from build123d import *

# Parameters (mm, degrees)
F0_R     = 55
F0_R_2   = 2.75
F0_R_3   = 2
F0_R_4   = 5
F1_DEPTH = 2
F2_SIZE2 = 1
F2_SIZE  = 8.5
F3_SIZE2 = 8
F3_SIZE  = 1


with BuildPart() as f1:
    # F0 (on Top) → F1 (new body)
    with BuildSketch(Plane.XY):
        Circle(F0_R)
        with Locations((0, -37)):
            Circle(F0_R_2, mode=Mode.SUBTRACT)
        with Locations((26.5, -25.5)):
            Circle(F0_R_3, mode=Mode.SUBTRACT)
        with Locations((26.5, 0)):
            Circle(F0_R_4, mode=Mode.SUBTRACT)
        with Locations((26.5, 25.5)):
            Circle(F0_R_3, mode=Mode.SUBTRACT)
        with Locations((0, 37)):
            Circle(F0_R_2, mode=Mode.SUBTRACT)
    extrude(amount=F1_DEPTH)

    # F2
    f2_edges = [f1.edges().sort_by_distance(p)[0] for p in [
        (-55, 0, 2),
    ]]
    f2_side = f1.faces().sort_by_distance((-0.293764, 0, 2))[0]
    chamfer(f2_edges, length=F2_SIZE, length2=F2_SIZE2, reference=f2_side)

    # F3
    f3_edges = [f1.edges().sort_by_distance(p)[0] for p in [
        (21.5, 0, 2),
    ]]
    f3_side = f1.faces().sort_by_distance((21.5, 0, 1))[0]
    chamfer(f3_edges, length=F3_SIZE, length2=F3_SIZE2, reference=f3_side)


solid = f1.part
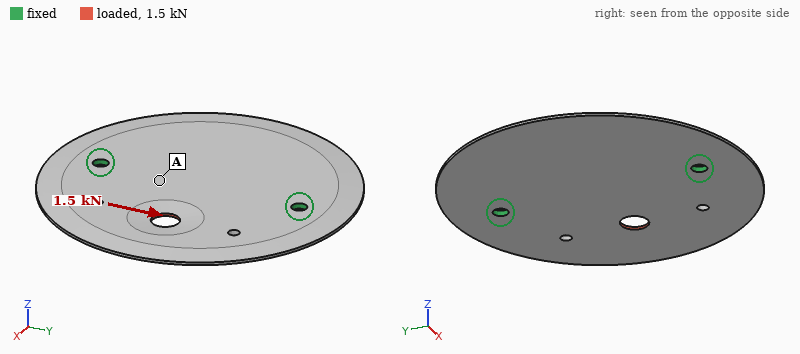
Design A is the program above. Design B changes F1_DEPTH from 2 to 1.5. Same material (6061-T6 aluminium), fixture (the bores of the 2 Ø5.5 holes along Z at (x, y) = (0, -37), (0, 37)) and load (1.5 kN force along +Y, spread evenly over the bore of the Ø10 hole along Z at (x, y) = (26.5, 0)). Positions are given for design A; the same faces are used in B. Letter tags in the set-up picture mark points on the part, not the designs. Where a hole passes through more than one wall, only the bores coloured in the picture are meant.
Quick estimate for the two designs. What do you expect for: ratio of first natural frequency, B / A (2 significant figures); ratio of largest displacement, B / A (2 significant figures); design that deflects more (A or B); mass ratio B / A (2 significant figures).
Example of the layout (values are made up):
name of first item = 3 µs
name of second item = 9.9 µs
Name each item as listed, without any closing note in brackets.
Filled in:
ratio of first natural frequency, B / A = 0.77
ratio of largest displacement, B / A = 2.4
design that deflects more = B
mass ratio B / A = 0.73
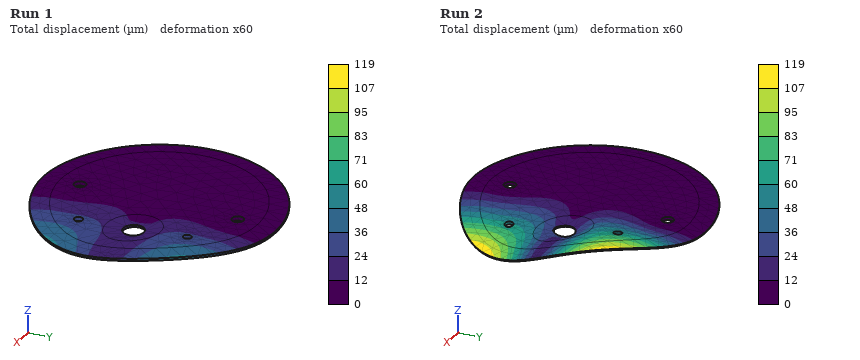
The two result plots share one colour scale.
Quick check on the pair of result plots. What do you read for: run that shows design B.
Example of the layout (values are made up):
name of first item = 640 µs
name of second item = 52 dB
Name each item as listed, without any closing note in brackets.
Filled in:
run that shows design B = Run 2
